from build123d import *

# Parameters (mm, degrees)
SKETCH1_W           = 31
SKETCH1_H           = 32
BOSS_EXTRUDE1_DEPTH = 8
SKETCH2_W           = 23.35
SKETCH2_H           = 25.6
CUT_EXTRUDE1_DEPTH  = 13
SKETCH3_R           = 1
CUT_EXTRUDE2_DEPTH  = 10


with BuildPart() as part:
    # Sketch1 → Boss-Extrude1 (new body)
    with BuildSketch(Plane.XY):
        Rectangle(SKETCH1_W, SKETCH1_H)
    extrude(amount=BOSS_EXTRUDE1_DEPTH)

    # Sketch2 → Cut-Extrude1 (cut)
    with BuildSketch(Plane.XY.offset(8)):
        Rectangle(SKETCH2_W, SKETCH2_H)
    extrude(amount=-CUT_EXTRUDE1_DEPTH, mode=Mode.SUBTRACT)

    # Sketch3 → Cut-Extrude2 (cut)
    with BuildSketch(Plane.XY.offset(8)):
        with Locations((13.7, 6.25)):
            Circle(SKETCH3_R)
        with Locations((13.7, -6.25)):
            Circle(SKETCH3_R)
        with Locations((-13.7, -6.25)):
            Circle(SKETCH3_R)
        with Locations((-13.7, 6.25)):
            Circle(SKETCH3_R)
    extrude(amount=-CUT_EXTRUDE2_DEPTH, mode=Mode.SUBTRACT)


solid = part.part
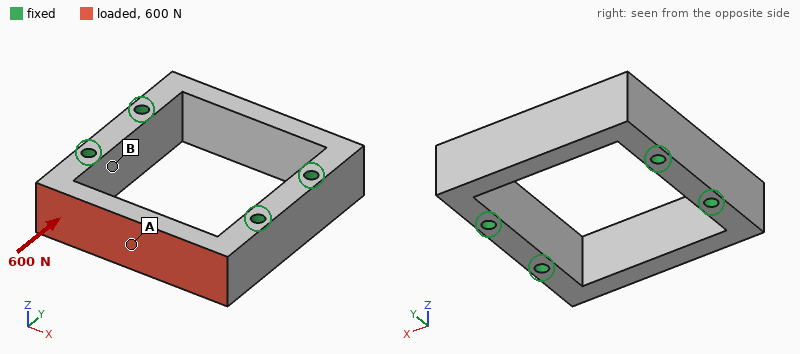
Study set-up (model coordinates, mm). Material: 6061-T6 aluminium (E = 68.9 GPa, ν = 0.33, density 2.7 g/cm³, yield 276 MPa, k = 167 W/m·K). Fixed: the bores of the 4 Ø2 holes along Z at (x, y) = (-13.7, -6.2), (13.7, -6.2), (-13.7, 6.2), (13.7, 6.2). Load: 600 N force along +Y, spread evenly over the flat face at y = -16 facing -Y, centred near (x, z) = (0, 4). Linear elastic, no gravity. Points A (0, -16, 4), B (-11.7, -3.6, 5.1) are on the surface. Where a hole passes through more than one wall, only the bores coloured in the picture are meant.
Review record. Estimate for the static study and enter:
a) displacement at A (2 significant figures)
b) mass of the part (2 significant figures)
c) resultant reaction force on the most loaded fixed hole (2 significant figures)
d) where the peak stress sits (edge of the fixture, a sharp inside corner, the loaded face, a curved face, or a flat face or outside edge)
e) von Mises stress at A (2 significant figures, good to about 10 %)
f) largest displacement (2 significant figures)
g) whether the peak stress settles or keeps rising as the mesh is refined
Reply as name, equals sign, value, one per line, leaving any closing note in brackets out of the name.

displacement at A = 23 µm
mass of the part = 8.2 g
resultant reaction force on the most loaded fixed hole = 350 N
where the peak stress sits = a sharp inside corner
von Mises stress at A = 50 MPa
largest displacement = 24 µm
whether the peak stress settles or keeps rising as the mesh is refined = keeps rising
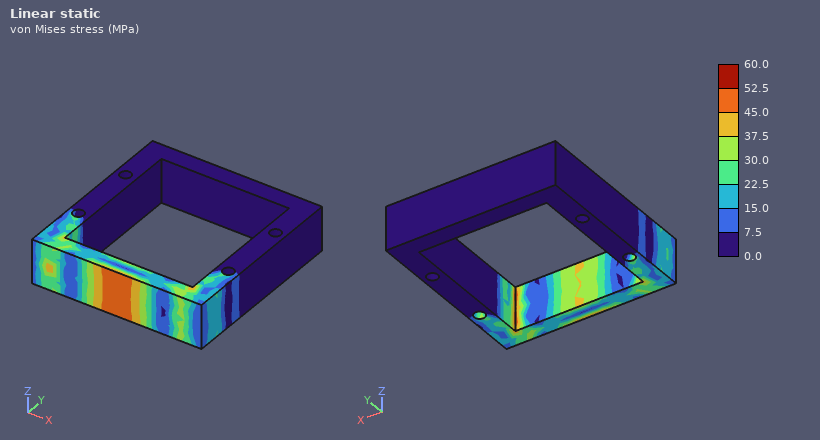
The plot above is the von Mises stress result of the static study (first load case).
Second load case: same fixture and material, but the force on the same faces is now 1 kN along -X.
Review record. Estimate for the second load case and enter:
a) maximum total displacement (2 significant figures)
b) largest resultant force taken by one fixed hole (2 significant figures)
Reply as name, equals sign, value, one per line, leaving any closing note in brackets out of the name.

maximum total displacement = 31 µm
largest resultant force taken by one fixed hole = 550 N
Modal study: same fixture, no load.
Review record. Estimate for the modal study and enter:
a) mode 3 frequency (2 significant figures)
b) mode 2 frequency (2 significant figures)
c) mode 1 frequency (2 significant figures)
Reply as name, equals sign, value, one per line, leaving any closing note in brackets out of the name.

mode 3 frequency = 20 kHz
mode 2 frequency = 20 kHz
mode 1 frequency = 20 kHz
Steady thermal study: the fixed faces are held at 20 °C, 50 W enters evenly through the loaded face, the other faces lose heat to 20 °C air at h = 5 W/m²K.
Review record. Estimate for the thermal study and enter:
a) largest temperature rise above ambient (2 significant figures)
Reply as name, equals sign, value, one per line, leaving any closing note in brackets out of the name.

largest temperature rise above ambient = 65 K
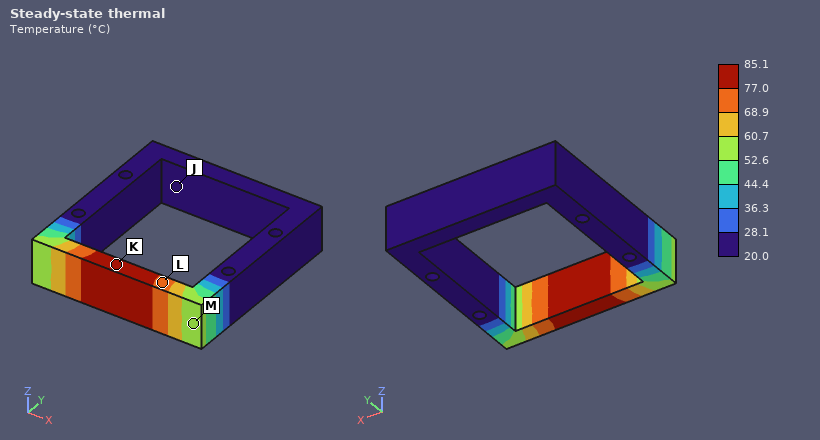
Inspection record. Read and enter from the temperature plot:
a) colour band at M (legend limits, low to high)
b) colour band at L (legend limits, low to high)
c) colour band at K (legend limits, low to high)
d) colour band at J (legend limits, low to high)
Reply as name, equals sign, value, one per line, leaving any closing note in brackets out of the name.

colour band at M = 52.6 to 60.7 °C
colour band at L = 68.9 to 77.0 °C
colour band at K = 77.0 to 85.1 °C
colour band at J = 20.0 to 28.1 °C
